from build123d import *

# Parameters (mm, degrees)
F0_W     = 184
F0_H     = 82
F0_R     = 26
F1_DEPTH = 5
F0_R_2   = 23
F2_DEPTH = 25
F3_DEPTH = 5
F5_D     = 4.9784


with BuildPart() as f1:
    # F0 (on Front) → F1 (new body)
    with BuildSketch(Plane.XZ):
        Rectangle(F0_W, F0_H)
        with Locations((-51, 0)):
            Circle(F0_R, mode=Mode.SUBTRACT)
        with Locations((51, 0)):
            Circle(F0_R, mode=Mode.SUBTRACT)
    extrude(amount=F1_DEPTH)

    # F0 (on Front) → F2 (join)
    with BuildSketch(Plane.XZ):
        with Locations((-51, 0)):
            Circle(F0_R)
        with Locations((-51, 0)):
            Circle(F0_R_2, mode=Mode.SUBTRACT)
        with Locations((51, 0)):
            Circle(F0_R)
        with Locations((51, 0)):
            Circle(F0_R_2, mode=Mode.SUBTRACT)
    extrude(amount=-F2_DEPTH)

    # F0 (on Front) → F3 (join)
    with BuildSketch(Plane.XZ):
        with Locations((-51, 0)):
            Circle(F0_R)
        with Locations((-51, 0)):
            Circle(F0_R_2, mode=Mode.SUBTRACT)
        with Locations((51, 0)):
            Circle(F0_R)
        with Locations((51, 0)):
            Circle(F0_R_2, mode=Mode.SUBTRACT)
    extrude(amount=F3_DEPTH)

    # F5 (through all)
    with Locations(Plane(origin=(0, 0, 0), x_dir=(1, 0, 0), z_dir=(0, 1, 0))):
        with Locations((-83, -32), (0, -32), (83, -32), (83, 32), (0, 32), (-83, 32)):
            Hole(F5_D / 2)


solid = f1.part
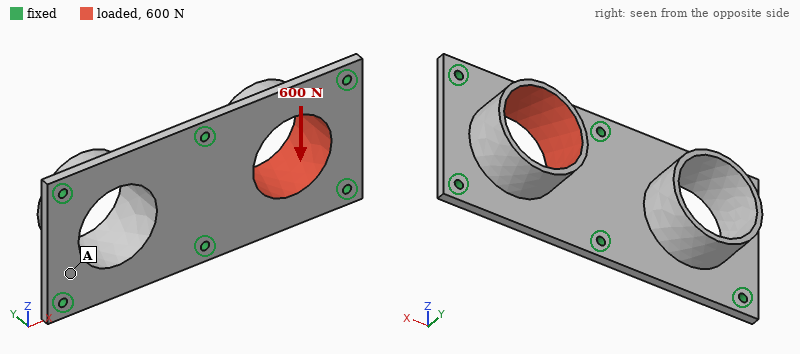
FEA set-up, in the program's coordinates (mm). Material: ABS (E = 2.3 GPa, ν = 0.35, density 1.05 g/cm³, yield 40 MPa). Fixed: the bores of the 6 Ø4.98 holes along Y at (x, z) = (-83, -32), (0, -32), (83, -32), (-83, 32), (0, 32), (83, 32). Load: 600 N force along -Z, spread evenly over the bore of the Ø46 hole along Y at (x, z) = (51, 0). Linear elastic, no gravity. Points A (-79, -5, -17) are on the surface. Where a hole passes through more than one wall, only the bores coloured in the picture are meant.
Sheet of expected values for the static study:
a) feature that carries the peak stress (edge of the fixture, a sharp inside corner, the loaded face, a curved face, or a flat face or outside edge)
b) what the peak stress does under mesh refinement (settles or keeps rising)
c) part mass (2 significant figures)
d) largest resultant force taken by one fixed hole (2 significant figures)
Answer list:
edge of the fixture
keeps rising
85 g
190 N
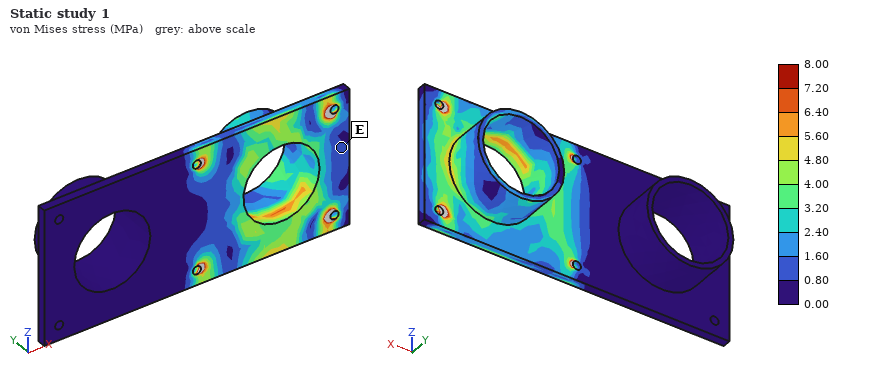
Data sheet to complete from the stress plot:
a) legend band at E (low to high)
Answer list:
0.80 to 1.60 MPa
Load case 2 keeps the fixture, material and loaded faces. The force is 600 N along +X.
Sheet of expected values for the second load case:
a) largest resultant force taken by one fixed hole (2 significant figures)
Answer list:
170 N
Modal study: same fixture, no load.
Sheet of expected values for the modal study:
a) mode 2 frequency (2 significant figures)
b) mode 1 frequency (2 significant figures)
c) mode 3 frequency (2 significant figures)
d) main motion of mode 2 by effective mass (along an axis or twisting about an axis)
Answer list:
970 Hz
920 Hz
1100 Hz
along Y
